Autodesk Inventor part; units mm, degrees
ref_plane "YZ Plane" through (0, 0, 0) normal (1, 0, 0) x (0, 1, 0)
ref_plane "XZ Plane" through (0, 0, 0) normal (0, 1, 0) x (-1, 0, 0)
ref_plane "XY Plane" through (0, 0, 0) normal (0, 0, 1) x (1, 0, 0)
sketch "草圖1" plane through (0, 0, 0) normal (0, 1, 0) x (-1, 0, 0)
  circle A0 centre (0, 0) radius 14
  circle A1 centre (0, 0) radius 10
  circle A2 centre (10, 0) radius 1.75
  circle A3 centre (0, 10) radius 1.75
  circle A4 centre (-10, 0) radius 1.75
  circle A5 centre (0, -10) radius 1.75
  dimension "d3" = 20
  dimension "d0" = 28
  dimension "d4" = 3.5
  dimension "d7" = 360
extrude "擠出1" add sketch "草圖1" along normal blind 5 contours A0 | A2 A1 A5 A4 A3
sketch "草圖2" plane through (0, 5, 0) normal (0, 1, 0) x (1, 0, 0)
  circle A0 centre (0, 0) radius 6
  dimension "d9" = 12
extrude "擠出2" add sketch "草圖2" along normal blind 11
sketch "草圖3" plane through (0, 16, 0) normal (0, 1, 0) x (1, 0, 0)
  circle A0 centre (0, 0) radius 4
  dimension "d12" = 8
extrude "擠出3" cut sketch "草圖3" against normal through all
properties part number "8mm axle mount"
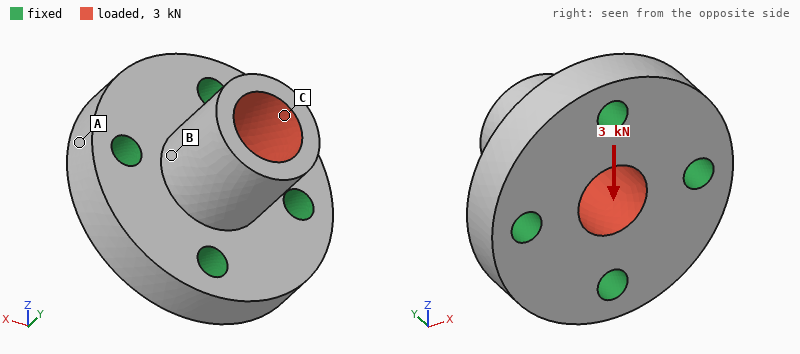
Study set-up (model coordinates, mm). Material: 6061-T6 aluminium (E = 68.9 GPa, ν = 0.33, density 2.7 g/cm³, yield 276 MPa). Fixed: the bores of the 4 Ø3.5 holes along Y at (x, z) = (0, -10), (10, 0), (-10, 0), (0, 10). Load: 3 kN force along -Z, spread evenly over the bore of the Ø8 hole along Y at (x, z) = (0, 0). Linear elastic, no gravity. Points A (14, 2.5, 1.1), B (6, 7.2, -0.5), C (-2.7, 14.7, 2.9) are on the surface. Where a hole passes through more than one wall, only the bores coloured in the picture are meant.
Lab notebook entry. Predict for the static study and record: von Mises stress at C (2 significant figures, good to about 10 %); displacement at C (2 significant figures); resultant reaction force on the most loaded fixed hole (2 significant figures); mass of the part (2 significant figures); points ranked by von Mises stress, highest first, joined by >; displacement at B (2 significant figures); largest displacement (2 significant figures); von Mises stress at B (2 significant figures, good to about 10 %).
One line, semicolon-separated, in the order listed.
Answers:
24 MPa; 28 µm; 1.3 kN; 9.0 g; B > C > A; 8.7 µm; 32 µm; 56 MPa
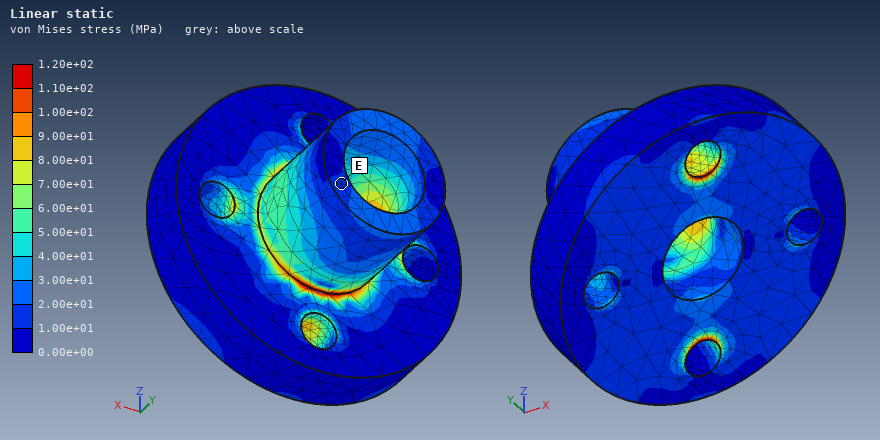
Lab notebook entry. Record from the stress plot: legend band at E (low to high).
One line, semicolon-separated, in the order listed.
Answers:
1.00e+01 to 2.00e+01 MPa
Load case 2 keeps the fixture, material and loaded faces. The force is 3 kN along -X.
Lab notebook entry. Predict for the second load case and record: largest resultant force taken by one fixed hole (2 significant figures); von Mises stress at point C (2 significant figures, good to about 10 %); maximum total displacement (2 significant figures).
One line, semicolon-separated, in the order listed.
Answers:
1.3 kN; 25 MPa; 32 µm
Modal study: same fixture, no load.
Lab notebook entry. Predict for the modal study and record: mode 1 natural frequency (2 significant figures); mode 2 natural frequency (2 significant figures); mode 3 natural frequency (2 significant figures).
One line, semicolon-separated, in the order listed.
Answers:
34 kHz; 34 kHz; 55 kHz
